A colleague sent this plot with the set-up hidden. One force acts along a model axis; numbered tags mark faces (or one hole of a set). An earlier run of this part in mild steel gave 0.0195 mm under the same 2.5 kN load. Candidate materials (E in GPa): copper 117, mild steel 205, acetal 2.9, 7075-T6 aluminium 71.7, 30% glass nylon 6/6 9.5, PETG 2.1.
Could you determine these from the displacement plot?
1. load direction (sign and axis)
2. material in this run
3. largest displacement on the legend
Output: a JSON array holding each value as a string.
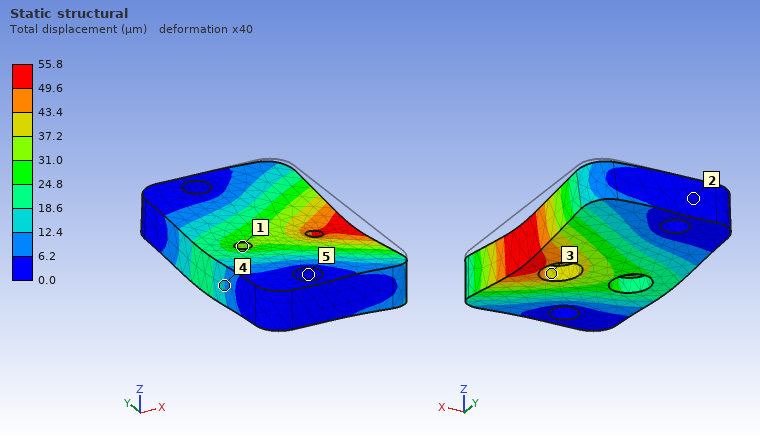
["-Z", "7075-T6 aluminium", "55.8 µm"]
